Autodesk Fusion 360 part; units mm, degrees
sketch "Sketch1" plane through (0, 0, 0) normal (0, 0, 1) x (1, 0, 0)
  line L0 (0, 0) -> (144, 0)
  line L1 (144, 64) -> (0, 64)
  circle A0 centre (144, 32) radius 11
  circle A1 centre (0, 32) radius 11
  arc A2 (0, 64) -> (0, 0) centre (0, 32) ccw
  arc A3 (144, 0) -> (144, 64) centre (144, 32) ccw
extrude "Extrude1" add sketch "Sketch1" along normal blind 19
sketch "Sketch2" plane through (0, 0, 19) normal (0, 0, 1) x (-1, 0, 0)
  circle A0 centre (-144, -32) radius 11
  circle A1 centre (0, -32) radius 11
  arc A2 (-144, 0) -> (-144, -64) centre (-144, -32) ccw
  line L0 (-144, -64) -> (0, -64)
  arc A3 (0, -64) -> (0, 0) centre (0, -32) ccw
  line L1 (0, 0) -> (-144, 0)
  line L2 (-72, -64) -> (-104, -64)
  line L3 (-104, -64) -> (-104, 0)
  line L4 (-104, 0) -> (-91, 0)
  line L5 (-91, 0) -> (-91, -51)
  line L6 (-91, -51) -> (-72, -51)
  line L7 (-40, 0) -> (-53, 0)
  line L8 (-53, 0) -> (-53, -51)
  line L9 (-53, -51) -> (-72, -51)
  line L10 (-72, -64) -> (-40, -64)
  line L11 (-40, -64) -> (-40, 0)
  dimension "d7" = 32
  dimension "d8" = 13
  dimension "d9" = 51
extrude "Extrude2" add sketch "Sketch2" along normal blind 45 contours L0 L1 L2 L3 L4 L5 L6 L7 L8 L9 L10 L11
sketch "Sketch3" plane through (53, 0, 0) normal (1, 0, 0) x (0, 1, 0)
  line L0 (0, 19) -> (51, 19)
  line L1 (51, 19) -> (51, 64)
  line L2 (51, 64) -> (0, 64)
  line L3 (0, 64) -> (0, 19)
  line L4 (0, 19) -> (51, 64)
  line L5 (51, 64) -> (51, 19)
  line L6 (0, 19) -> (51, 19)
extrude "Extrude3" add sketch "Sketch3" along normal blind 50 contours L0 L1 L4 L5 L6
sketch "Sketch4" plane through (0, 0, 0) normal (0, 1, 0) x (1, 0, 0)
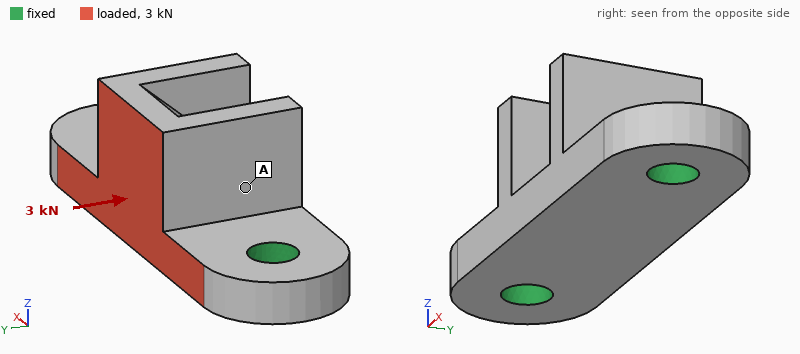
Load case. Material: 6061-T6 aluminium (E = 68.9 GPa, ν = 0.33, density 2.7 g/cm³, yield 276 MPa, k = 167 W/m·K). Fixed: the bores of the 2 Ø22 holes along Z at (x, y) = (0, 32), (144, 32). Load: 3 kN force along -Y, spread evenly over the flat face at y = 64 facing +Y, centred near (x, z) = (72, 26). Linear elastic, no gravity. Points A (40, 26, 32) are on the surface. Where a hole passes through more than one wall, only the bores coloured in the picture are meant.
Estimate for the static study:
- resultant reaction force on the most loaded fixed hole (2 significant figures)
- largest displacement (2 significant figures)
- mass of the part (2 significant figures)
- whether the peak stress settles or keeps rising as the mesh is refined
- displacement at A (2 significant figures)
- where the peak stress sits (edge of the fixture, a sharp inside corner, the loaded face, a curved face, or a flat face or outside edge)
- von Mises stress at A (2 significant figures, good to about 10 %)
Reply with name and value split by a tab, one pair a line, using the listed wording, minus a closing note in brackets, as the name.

resultant reaction force on the most loaded fixed hole	1.5 kN
largest displacement	20 µm
mass of the part	980 g
whether the peak stress settles or keeps rising as the mesh is refined	keeps rising
displacement at A	9.0 µm
where the peak stress sits	edge of the fixture
von Mises stress at A	1.6 MPa
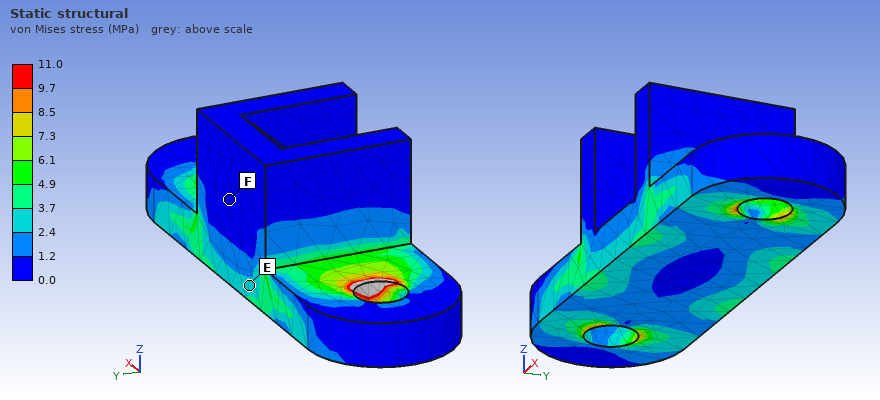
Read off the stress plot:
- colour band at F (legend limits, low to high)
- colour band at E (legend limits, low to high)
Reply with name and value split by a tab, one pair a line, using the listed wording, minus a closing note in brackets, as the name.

colour band at F	0.0 to 1.2 MPa
colour band at E	2.4 to 3.7 MPa
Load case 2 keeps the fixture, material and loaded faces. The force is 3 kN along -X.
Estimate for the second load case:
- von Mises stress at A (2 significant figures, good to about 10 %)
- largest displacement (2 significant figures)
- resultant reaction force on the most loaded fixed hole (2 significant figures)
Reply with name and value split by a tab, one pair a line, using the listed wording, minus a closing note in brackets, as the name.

von Mises stress at A	1.1 MPa
largest displacement	5.4 µm
resultant reaction force on the most loaded fixed hole	1.7 kN
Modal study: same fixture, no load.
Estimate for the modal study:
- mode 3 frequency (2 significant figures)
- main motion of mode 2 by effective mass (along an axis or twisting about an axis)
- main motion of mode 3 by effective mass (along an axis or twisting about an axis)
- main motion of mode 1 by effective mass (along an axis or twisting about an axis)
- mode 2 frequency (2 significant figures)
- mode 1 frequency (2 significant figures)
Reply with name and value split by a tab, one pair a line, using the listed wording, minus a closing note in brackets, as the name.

mode 3 frequency	5700 Hz
main motion of mode 2 by effective mass	along Z
main motion of mode 3 by effective mass	along X
main motion of mode 1 by effective mass	along Y
mode 2 frequency	4100 Hz
mode 1 frequency	2700 Hz
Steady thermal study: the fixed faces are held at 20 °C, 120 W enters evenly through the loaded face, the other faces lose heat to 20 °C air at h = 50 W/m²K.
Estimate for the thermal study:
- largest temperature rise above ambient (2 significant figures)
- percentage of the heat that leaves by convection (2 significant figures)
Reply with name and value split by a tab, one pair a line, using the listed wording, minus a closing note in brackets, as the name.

largest temperature rise above ambient	15 K
percentage of the heat that leaves by convection	11 %
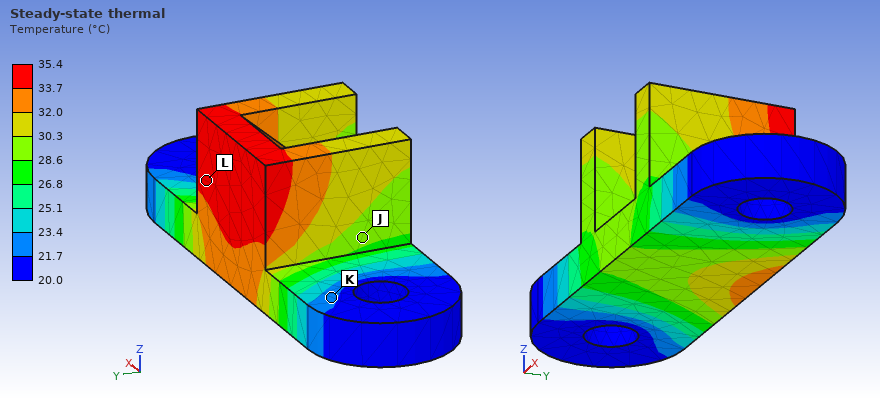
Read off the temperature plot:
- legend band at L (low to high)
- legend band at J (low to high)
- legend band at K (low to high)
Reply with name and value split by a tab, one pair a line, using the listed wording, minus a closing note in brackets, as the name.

legend band at L	33.7 to 35.4 °C
legend band at J	28.6 to 30.3 °C
legend band at K	21.7 to 23.4 °C
